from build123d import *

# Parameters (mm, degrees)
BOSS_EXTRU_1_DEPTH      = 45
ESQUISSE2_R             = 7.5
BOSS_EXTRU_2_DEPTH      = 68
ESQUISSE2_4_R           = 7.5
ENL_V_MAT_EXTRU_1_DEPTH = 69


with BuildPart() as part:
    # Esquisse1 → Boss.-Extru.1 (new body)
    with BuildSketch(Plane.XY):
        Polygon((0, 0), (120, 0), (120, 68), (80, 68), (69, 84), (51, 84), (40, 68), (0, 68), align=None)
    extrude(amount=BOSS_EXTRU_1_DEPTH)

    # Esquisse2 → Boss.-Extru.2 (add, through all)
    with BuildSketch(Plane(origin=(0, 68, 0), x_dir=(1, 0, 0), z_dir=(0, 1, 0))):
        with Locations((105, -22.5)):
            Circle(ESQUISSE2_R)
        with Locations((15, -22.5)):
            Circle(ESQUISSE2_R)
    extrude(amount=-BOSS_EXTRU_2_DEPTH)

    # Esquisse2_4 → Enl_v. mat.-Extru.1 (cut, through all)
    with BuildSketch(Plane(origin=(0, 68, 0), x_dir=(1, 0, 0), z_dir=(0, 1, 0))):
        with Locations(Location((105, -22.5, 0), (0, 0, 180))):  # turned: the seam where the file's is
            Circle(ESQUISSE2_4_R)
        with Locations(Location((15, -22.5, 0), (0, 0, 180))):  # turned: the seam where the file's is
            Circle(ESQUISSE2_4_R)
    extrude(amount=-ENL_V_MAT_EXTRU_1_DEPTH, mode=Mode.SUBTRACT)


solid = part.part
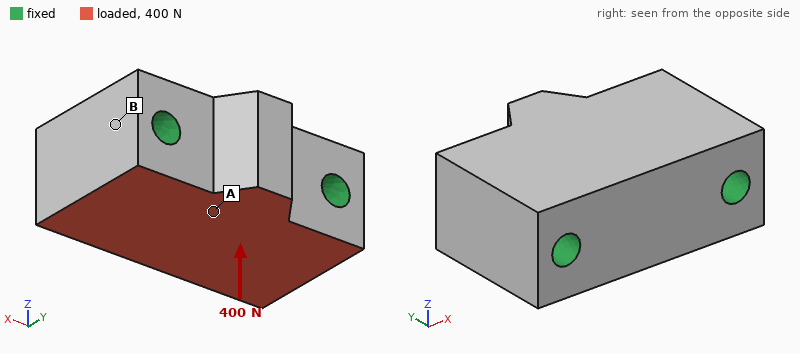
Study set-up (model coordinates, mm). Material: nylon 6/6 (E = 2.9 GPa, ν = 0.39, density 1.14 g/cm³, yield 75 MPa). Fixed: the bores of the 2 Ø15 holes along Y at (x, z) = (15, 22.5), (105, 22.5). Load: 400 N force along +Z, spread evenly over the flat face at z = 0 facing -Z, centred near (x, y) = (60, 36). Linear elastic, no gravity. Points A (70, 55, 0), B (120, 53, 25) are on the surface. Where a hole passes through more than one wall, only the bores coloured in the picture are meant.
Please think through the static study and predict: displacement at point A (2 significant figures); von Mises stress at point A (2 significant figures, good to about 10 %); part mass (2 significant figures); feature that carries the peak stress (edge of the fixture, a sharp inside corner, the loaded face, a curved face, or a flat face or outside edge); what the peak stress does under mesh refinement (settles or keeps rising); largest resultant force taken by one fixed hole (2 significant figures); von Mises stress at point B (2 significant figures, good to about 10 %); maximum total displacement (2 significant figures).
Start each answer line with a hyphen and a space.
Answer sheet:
- 2.1 µm
- 0.099 MPa
- 420 g
- edge of the fixture
- keeps rising
- 200 N
- 0.032 MPa
- 3.4 µm
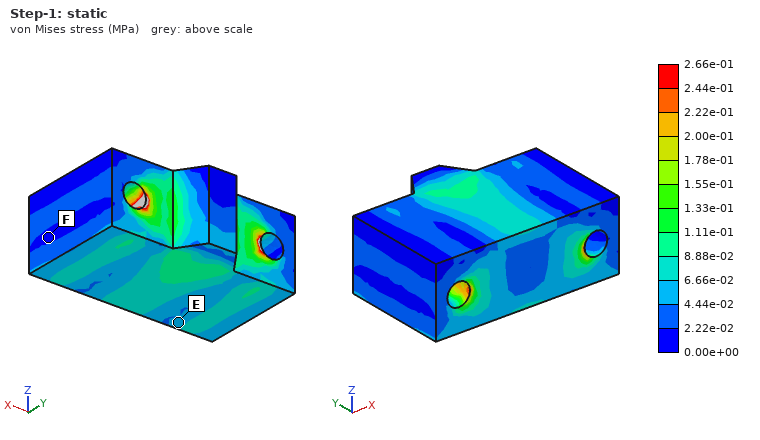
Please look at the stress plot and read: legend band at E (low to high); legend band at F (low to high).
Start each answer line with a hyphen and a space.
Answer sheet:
- 4.44e-02 to 6.66e-02 MPa
- 0.00e+00 to 2.22e-02 MPa
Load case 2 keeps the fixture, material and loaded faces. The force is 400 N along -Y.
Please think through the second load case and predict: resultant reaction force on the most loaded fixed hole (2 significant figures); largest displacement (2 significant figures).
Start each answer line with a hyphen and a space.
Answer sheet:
- 200 N
- 5.3 µm
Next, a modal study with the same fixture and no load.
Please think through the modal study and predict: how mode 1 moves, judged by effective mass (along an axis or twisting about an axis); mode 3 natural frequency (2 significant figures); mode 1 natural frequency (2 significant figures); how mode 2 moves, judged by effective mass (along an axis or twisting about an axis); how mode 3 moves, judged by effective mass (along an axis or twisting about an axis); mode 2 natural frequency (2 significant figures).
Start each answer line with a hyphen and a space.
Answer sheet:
- along Z
- 4700 Hz
- 3500 Hz
- along Z
- along Y
- 4400 Hz
